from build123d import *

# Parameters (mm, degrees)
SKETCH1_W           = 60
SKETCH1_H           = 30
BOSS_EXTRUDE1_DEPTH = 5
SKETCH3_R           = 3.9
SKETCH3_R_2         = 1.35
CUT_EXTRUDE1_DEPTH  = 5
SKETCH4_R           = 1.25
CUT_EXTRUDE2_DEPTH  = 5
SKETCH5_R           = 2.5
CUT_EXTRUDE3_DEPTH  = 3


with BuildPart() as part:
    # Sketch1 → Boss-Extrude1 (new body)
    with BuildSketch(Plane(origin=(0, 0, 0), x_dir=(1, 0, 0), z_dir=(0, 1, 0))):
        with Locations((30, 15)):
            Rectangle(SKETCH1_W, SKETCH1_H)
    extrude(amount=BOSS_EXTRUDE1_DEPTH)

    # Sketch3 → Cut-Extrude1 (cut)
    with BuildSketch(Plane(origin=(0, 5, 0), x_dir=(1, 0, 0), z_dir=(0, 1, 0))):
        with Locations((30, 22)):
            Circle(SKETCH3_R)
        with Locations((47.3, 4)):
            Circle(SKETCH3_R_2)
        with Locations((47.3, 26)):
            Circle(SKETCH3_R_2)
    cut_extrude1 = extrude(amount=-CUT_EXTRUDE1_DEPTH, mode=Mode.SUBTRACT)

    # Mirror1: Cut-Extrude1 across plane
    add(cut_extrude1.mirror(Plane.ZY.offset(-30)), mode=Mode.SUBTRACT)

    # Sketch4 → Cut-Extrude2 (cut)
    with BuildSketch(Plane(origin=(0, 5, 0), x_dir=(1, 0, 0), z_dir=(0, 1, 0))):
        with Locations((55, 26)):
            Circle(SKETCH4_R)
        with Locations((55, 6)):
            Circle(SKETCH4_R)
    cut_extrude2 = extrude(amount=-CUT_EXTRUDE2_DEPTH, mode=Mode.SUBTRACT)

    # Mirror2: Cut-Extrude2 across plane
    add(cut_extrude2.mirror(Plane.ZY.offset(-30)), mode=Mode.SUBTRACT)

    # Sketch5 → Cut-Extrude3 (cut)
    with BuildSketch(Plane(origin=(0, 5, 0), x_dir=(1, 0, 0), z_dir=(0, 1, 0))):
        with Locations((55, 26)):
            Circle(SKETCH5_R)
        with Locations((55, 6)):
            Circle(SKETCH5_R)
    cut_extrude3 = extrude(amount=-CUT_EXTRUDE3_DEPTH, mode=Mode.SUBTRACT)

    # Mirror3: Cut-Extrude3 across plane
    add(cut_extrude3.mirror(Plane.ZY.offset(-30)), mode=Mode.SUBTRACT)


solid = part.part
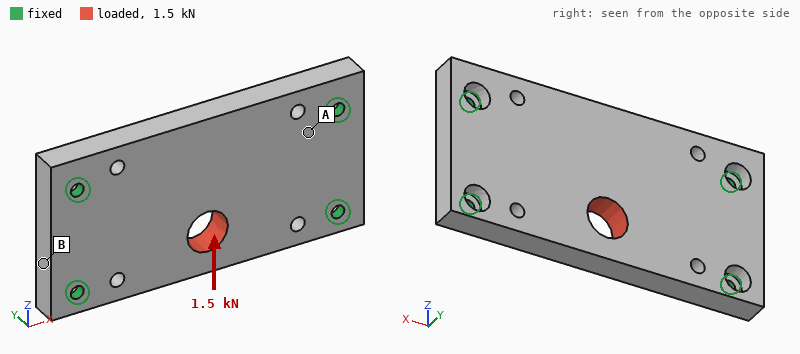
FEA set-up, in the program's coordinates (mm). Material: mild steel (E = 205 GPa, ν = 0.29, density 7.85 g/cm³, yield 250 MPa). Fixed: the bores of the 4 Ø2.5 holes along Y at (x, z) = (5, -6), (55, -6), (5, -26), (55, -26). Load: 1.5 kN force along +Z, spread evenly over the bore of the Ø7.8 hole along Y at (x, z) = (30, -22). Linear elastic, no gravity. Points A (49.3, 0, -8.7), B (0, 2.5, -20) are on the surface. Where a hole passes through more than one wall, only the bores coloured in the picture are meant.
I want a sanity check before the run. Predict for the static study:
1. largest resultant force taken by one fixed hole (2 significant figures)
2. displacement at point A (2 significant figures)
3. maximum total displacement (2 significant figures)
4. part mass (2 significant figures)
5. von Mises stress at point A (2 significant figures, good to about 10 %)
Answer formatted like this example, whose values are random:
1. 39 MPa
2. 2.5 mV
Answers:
1. 510 N
2. 0.96 µm
3. 3.7 µm
4. 66 g
5. 17 MPa
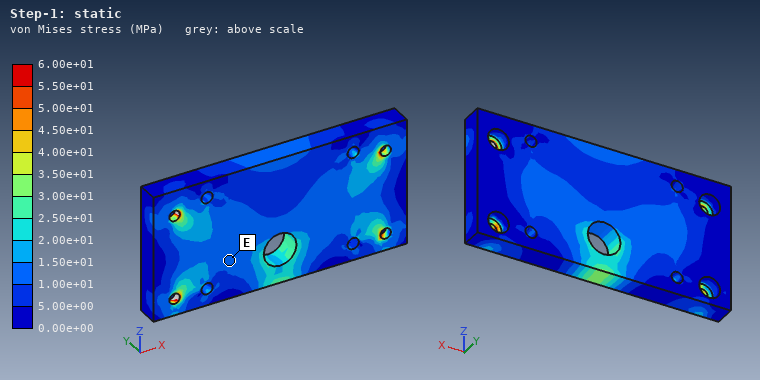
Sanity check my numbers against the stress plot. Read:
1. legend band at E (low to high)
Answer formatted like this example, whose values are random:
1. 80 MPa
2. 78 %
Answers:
1. 1.00e+01 to 1.50e+01 MPa
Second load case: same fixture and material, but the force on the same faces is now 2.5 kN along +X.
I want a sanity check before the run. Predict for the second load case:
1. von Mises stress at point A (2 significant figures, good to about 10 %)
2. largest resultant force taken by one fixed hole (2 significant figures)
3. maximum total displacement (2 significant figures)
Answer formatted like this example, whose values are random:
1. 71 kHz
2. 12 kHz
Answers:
1. 19 MPa
2. 700 N
3. 3.0 µm
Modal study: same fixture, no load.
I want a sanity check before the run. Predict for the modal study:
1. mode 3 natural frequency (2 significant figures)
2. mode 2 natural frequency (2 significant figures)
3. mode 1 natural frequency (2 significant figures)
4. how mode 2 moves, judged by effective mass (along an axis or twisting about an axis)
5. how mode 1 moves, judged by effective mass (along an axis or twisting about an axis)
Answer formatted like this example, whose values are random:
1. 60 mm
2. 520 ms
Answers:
1. 18 kHz
2. 12 kHz
3. 6800 Hz
4. twisting about X
5. along Y
